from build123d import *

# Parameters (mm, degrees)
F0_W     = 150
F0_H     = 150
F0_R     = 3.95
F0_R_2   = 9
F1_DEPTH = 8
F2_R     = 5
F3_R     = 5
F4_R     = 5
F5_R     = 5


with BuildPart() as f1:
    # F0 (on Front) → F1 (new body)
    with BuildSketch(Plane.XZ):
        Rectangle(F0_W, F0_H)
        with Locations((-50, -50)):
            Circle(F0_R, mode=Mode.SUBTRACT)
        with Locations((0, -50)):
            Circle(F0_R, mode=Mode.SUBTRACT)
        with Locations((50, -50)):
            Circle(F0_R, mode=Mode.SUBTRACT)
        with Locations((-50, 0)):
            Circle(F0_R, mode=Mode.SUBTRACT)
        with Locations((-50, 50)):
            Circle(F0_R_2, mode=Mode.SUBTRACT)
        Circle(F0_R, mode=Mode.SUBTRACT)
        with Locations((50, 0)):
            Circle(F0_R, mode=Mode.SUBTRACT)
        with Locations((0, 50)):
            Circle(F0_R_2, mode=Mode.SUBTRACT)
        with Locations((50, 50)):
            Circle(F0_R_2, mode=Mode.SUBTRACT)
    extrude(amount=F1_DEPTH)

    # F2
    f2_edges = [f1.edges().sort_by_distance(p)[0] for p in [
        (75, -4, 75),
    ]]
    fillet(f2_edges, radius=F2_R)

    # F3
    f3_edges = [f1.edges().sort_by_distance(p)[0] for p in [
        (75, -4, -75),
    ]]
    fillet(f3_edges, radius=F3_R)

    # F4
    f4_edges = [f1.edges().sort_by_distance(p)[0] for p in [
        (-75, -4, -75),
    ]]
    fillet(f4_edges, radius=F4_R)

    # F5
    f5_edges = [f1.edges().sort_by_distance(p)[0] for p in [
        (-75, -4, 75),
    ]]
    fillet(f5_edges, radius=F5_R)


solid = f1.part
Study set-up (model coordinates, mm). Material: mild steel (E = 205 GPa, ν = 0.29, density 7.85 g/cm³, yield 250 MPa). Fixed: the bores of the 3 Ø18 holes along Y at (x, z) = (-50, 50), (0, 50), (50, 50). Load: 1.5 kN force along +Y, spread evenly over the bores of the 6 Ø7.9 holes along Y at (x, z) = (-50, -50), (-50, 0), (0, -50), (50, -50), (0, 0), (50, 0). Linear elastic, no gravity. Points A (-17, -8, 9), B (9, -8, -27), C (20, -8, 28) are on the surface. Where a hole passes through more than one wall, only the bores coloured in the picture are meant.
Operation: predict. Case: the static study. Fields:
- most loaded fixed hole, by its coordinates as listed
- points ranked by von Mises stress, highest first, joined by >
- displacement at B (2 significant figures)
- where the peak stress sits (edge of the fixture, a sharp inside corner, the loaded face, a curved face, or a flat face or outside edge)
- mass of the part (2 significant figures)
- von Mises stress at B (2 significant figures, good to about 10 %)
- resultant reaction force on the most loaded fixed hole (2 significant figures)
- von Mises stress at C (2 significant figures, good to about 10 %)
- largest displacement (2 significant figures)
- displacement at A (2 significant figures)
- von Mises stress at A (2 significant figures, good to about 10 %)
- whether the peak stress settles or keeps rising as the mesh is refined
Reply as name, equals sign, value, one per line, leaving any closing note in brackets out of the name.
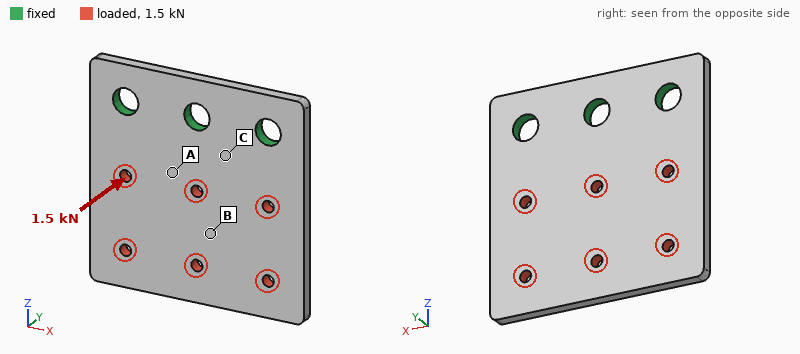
most loaded fixed hole, by its coordinates as listed = (0, 50)
points ranked by von Mises stress, highest first, joined by > = C > A > B
displacement at B = 0.13 mm
where the peak stress sits = edge of the fixture
mass of the part = 1.3 kg
von Mises stress at B = 10 MPa
resultant reaction force on the most loaded fixed hole = 590 N
von Mises stress at C = 45 MPa
largest displacement = 0.28 mm
displacement at A = 0.043 mm
von Mises stress at A = 30 MPa
whether the peak stress settles or keeps rising as the mesh is refined = keeps rising
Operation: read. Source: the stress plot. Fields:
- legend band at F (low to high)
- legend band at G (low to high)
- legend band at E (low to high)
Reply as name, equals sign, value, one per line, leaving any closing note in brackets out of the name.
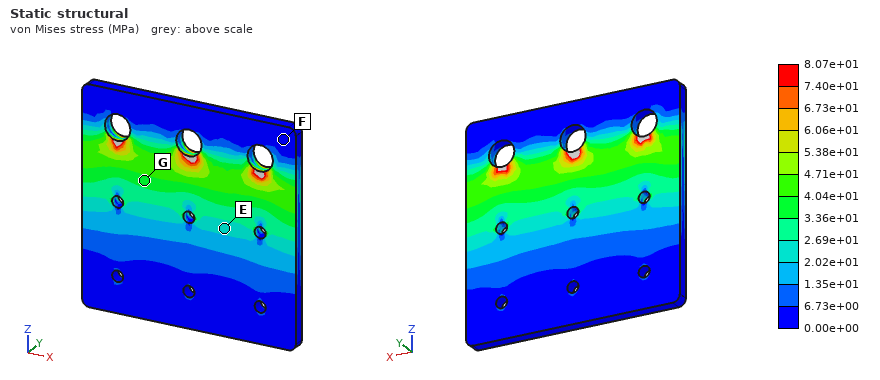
legend band at F = 0.00e+00 to 6.73e+00 MPa
legend band at G = 3.36e+01 to 4.04e+01 MPa
legend band at E = 2.02e+01 to 2.69e+01 MPa
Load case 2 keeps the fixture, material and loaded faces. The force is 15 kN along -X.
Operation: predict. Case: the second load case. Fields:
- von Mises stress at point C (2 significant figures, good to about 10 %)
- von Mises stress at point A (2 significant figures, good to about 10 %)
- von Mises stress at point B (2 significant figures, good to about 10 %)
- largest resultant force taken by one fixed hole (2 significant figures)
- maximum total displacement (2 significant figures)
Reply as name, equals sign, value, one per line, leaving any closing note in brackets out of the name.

von Mises stress at point C = 28 MPa
von Mises stress at point A = 28 MPa
von Mises stress at point B = 17 MPa
largest resultant force taken by one fixed hole = 11 kN
maximum total displacement = 27 µm
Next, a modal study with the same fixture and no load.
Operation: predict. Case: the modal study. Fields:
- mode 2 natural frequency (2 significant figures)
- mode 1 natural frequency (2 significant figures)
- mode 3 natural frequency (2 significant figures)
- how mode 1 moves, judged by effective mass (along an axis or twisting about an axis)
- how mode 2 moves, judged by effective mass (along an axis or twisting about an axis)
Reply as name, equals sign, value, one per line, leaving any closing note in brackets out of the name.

mode 2 natural frequency = 960 Hz
mode 1 natural frequency = 470 Hz
mode 3 natural frequency = 2400 Hz
how mode 1 moves, judged by effective mass = along Y
how mode 2 moves, judged by effective mass = twisting about Z
